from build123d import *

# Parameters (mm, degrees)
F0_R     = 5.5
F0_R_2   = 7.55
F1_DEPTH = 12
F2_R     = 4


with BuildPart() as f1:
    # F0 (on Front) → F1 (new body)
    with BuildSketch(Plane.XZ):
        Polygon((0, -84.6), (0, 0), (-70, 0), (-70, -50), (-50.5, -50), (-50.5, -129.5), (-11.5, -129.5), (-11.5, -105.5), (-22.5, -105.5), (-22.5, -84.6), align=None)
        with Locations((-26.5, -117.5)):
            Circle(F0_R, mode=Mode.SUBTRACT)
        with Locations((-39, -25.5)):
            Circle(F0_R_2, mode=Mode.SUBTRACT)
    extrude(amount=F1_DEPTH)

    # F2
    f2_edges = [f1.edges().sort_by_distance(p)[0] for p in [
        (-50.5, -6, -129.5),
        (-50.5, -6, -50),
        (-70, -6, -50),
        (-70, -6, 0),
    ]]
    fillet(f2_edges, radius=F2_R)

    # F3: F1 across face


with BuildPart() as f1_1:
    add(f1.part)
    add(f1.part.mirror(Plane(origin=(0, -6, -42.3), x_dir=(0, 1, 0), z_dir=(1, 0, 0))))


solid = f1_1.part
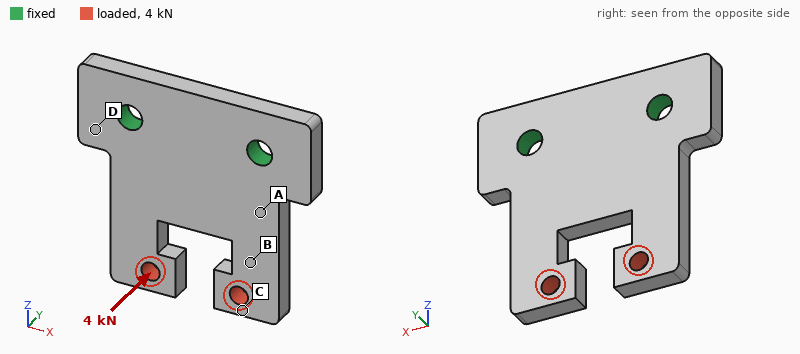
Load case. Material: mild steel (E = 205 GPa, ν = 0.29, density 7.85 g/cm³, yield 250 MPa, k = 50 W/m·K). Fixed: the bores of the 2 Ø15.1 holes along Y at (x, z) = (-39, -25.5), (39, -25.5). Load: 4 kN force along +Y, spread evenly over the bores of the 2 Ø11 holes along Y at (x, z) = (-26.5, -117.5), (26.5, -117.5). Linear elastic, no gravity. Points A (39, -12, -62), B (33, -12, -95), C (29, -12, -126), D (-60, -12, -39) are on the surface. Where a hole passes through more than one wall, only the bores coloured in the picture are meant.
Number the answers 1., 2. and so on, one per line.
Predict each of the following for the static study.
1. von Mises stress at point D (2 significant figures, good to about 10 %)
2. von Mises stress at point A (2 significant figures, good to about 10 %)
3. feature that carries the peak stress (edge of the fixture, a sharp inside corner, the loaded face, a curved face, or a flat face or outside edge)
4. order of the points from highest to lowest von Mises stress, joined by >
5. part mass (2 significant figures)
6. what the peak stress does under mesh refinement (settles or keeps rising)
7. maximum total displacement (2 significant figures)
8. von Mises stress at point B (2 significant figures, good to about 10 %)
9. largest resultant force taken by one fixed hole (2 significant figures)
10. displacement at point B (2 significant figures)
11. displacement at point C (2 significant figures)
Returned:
1. 47 MPa
2. 100 MPa
3. edge of the fixture
4. A > B > D > C
5. 1.2 kg
6. keeps rising
7. 0.45 mm
8. 75 MPa
9. 2.0 kN
10. 0.21 mm
11. 0.41 mm
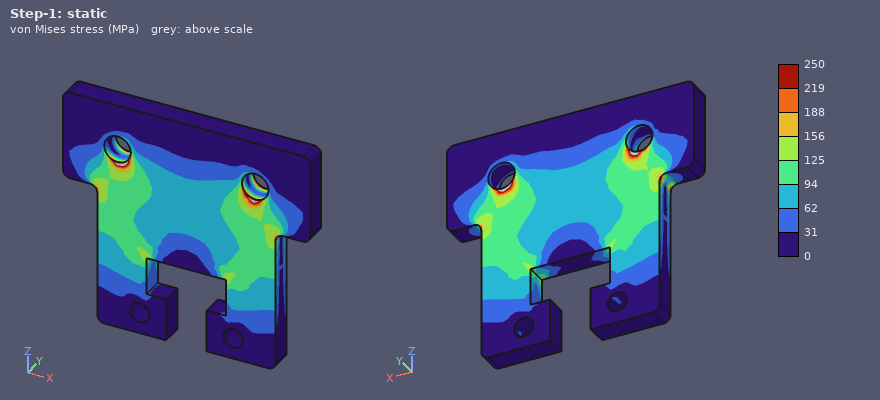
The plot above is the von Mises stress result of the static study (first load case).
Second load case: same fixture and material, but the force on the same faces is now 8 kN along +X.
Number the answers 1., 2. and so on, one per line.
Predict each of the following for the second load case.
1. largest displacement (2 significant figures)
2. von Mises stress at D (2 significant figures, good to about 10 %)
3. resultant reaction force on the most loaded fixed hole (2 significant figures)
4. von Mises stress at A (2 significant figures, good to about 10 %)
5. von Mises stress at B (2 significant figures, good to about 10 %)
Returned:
1. 69 µm
2. 7.1 MPa
3. 9.4 kN
4. 21 MPa
5. 35 MPa
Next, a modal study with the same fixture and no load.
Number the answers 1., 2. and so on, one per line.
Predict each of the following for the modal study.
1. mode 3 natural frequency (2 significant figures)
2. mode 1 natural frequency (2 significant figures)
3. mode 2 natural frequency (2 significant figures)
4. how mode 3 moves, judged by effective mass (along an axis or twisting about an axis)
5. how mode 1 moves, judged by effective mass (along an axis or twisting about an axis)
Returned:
1. 4400 Hz
2. 1100 Hz
3. 1600 Hz
4. along X
5. along Y
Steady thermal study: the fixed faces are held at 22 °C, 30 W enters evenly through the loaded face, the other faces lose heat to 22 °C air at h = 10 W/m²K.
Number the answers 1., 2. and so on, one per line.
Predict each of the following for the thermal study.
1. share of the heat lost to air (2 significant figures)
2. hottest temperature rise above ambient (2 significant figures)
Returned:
1. 20 %
2. 61 K
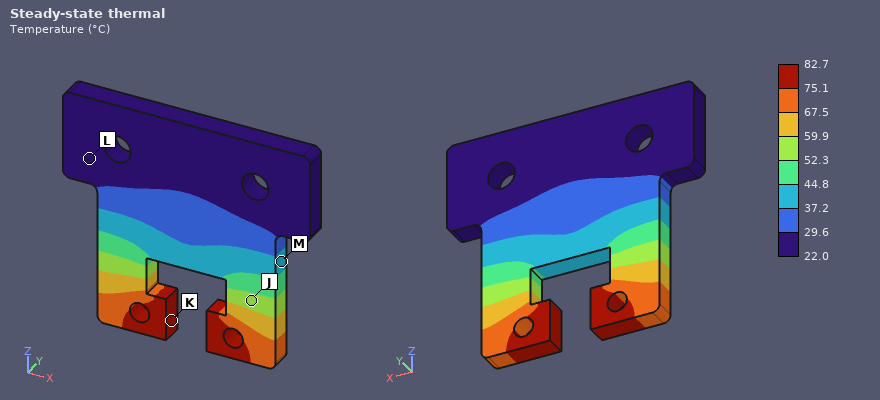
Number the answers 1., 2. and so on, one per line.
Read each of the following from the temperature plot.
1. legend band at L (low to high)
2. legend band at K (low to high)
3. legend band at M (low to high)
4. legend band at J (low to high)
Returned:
1. 22.0 to 29.6 °C
2. 75.1 to 82.7 °C
3. 37.2 to 44.8 °C
4. 52.3 to 59.9 °C
